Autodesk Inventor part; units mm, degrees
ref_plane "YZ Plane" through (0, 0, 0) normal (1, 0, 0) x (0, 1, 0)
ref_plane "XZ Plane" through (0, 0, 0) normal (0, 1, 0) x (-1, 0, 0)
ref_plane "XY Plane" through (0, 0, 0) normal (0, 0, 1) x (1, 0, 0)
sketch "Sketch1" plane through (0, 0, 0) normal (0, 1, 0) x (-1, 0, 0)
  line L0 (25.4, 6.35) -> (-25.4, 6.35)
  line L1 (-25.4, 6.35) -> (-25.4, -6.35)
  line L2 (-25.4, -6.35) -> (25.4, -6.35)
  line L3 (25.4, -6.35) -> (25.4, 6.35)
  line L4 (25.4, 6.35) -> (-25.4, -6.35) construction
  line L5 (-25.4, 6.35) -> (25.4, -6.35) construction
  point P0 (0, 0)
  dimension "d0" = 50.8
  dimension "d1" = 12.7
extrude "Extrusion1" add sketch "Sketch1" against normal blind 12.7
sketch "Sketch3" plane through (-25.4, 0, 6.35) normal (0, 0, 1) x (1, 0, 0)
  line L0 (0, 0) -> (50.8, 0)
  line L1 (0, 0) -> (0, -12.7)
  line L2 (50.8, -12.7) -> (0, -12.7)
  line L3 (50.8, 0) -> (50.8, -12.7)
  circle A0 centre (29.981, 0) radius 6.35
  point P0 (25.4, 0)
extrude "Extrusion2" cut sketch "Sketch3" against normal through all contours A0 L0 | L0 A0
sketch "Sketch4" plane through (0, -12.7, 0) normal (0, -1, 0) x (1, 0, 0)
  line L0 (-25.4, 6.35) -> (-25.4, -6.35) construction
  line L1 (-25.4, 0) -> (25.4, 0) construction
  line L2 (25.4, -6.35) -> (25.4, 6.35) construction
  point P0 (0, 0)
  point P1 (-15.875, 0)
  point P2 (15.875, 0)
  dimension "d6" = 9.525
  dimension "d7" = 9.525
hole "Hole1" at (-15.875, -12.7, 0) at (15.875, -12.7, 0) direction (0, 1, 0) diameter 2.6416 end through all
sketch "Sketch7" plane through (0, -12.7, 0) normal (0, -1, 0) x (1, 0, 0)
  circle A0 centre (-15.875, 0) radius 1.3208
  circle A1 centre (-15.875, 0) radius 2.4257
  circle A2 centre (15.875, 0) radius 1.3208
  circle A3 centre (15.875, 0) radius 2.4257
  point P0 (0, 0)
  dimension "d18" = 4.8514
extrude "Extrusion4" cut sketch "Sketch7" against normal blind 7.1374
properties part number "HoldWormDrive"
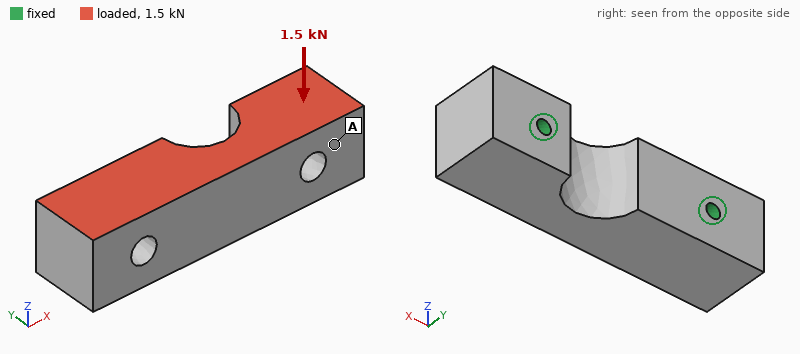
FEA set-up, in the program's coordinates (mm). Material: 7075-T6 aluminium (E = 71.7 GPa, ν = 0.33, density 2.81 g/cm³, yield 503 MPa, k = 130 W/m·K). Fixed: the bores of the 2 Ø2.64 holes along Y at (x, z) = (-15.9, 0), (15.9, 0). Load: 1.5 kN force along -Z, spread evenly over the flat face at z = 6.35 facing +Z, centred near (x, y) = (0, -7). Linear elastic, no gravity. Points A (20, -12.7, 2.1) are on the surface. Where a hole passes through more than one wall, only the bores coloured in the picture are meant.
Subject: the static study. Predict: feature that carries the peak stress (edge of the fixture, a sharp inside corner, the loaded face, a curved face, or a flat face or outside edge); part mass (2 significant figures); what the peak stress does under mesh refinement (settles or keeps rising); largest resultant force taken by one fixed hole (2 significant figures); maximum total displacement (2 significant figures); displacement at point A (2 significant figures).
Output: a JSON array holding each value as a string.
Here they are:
["edge of the fixture", "20 g", "keeps rising", "780 N", "9.5 µm", "6.5 µm"]
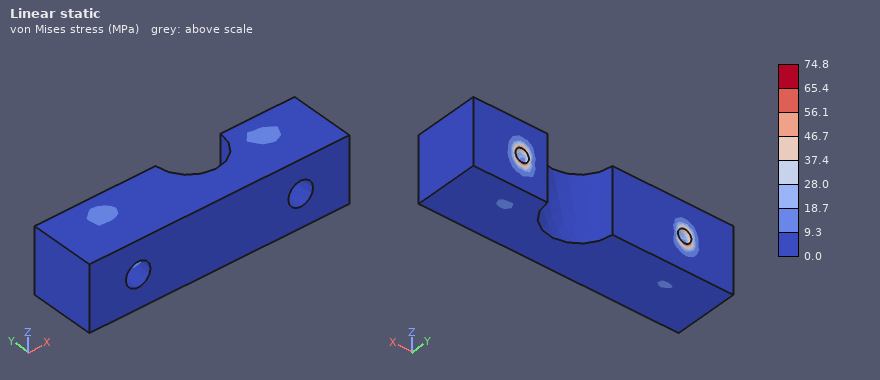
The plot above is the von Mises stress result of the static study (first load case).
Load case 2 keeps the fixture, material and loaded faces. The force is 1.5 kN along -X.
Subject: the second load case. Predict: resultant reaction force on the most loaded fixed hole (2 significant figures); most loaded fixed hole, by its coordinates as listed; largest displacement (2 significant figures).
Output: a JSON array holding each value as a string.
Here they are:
["920 N", "(-15.9, 0)", "6.4 µm"]
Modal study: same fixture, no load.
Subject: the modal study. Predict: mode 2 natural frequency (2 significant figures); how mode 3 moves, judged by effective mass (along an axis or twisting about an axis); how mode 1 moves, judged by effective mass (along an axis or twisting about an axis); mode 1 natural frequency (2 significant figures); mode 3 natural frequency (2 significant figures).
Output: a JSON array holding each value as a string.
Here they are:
["22 kHz", "twisting about Y", "along Z", "16 kHz", "24 kHz"]
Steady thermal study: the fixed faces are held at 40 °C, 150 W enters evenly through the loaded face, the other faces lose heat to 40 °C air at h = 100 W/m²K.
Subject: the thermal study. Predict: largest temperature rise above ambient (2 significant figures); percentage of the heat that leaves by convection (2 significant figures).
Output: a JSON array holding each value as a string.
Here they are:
["45 K", "4.2 %"]
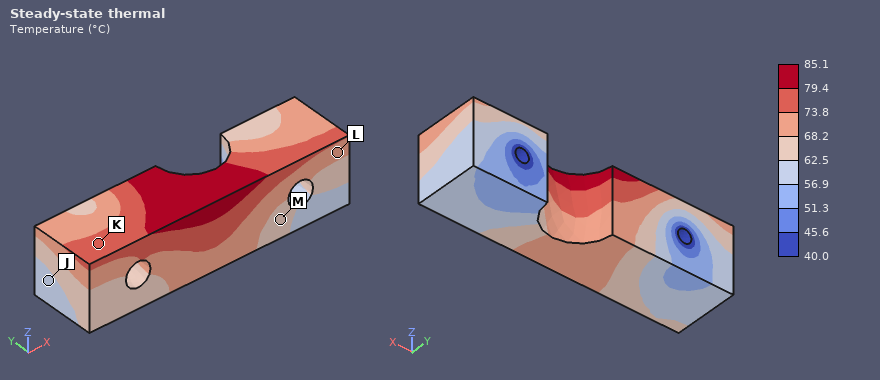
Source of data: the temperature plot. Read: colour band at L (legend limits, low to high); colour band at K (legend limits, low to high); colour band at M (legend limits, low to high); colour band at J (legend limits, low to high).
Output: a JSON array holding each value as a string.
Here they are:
["68.2 to 73.8 °C", "73.8 to 79.4 °C", "62.5 to 68.2 °C", "56.9 to 62.5 °C"]
